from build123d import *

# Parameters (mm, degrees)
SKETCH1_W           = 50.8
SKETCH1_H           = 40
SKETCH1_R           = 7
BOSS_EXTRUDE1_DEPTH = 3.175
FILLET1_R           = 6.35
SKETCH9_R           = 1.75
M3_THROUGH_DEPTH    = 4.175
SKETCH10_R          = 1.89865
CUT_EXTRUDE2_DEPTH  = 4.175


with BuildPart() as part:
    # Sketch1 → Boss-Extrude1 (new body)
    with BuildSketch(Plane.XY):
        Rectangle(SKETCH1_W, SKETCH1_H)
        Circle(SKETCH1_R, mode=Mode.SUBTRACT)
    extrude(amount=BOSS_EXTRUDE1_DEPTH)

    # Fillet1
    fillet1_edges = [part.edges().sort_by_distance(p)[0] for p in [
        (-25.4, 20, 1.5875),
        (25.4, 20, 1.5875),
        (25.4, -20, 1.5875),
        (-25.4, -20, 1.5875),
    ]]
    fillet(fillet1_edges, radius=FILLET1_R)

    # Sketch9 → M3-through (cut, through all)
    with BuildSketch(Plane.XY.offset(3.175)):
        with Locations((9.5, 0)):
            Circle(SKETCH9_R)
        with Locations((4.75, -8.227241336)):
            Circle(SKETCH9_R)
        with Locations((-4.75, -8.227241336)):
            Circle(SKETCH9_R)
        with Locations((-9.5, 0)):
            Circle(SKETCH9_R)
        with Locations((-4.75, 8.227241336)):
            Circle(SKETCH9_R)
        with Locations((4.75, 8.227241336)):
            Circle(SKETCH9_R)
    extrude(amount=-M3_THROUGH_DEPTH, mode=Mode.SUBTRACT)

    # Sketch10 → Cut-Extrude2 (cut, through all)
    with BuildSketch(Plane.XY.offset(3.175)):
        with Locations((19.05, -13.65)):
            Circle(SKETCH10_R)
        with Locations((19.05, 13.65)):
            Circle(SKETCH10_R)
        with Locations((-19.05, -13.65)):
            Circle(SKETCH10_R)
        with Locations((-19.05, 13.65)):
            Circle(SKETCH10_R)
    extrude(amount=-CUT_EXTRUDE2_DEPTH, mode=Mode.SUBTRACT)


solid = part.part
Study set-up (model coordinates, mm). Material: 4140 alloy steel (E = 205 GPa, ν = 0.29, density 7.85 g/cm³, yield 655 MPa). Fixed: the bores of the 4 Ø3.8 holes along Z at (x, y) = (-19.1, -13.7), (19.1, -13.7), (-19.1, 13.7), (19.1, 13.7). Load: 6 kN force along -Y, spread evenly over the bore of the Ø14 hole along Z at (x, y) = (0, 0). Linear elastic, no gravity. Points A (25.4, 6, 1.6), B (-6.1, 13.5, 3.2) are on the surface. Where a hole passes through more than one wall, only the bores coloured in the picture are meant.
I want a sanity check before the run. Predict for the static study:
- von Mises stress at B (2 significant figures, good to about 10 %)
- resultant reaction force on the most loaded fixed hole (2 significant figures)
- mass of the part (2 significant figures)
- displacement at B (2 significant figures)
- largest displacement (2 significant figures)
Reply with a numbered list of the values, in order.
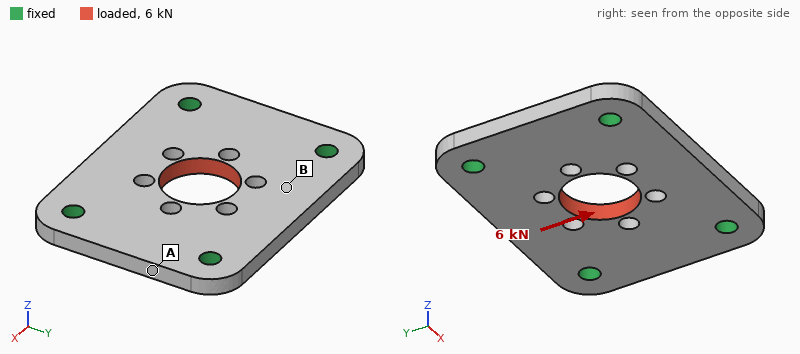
1. 41 MPa
2. 1.7 kN
3. 43 g
4. 5.5 µm
5. 9.4 µm
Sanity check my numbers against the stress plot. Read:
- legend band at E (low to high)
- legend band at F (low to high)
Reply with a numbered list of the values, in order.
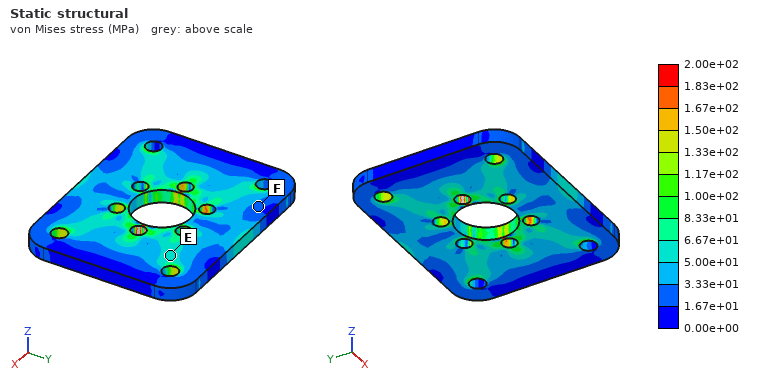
1. 5.00e+01 to 6.67e+01 MPa
2. 1.67e+01 to 3.33e+01 MPa
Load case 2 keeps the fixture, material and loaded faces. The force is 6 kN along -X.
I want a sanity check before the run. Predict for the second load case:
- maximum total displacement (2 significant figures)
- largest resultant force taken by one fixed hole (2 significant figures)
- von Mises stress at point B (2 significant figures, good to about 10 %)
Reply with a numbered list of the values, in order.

1. 6.7 µm
2. 1.6 kN
3. 34 MPa
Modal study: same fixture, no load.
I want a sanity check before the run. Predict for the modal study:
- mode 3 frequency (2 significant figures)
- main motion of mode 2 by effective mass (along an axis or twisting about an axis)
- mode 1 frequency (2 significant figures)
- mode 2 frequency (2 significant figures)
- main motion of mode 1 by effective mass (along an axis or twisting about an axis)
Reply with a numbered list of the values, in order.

1. 17 kHz
2. twisting about X
3. 11 kHz
4. 13 kHz
5. along Z
